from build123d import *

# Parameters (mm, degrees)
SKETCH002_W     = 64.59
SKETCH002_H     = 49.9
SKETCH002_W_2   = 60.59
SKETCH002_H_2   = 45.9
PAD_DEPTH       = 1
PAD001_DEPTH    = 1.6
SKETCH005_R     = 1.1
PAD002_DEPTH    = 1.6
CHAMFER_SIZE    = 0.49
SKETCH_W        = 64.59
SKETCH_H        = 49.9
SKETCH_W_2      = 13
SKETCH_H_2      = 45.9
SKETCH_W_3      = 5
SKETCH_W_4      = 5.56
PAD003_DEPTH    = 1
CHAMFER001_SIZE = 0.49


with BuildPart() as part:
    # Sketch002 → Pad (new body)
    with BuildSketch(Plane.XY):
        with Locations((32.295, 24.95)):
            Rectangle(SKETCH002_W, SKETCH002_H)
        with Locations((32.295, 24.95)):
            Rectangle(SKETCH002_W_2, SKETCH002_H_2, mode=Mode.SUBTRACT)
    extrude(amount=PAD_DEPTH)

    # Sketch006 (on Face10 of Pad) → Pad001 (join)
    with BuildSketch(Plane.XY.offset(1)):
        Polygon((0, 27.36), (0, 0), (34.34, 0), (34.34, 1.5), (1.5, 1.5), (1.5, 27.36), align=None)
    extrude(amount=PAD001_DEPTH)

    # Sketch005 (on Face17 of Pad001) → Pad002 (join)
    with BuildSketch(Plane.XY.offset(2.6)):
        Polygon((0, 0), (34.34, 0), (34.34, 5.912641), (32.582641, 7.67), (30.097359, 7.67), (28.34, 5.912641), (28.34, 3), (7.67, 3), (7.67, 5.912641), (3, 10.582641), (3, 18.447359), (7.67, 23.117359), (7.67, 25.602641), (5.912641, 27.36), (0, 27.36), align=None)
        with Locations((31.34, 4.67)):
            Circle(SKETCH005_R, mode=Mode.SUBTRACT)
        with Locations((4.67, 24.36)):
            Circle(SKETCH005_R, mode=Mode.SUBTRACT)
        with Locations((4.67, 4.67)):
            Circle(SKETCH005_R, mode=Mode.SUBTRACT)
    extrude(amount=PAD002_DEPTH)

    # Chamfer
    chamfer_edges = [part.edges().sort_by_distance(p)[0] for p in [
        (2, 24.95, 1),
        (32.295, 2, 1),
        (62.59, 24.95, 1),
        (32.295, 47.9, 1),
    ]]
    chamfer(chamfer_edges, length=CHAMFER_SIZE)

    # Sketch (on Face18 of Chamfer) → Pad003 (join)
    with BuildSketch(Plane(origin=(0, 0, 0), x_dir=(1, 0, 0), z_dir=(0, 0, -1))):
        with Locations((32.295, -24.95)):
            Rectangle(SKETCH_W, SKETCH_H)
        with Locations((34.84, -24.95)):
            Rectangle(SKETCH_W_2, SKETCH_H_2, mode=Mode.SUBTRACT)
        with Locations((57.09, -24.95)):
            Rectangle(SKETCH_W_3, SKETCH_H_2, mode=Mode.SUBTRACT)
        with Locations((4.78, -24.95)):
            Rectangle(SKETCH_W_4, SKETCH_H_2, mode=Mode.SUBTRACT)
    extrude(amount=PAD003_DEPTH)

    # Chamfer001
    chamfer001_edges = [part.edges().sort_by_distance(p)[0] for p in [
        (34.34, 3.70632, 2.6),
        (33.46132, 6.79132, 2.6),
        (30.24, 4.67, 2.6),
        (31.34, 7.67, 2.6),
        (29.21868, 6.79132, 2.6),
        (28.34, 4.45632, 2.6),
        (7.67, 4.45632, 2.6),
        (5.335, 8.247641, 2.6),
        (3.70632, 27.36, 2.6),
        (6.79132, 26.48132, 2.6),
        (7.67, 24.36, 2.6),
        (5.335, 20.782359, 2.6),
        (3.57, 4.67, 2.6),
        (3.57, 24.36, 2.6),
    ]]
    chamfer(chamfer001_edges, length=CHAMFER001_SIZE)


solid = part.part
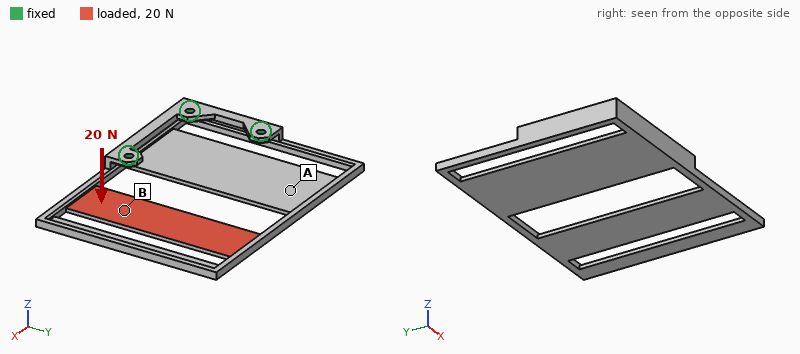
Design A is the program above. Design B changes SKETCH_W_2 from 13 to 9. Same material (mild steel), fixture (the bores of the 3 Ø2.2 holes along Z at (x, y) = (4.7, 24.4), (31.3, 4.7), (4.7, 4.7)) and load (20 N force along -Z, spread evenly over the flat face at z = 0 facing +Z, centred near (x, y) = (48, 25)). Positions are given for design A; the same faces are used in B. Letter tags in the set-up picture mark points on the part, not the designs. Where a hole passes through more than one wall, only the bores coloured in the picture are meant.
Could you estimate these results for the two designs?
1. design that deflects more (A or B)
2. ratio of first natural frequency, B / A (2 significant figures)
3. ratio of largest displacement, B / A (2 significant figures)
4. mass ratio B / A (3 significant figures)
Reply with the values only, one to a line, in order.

A
1.0
0.89
1.06
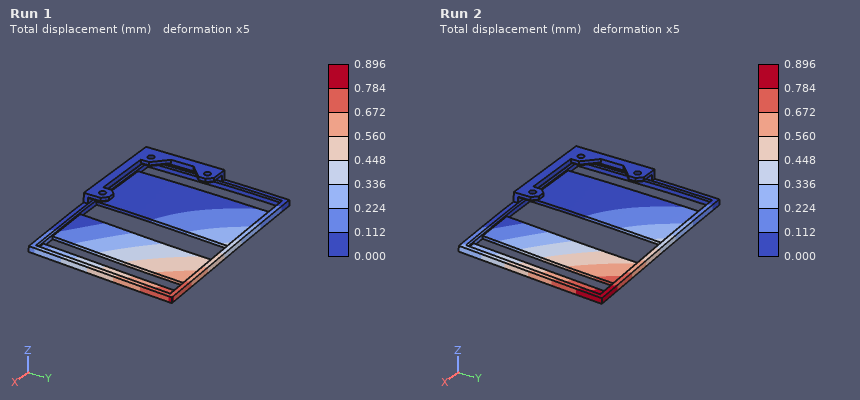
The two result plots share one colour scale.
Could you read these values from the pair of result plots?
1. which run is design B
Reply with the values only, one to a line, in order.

Run 1
